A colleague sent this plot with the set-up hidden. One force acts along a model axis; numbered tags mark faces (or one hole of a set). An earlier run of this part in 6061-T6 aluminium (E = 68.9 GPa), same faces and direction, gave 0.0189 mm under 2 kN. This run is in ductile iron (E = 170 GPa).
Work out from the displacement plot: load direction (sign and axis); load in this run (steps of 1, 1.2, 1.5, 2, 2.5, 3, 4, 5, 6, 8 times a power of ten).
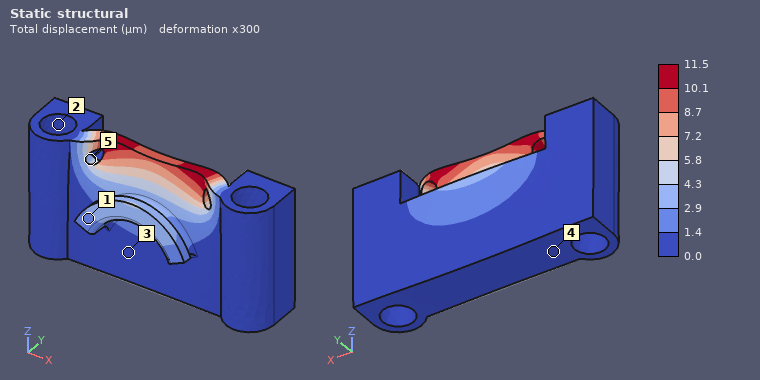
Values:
+Y
3 kN
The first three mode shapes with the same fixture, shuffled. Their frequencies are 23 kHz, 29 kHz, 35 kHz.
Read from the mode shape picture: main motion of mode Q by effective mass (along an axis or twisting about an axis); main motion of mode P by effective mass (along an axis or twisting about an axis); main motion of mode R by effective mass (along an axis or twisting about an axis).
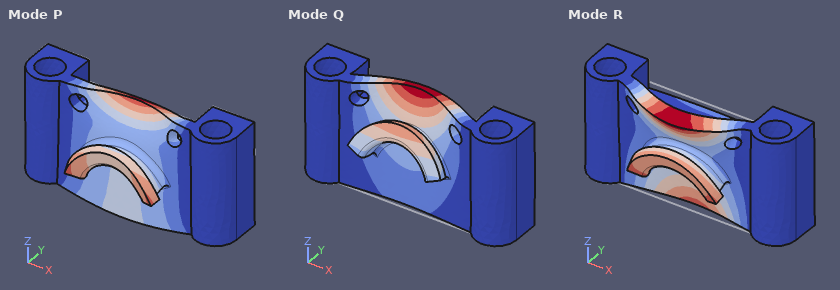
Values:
along Y
along Z
along Y
